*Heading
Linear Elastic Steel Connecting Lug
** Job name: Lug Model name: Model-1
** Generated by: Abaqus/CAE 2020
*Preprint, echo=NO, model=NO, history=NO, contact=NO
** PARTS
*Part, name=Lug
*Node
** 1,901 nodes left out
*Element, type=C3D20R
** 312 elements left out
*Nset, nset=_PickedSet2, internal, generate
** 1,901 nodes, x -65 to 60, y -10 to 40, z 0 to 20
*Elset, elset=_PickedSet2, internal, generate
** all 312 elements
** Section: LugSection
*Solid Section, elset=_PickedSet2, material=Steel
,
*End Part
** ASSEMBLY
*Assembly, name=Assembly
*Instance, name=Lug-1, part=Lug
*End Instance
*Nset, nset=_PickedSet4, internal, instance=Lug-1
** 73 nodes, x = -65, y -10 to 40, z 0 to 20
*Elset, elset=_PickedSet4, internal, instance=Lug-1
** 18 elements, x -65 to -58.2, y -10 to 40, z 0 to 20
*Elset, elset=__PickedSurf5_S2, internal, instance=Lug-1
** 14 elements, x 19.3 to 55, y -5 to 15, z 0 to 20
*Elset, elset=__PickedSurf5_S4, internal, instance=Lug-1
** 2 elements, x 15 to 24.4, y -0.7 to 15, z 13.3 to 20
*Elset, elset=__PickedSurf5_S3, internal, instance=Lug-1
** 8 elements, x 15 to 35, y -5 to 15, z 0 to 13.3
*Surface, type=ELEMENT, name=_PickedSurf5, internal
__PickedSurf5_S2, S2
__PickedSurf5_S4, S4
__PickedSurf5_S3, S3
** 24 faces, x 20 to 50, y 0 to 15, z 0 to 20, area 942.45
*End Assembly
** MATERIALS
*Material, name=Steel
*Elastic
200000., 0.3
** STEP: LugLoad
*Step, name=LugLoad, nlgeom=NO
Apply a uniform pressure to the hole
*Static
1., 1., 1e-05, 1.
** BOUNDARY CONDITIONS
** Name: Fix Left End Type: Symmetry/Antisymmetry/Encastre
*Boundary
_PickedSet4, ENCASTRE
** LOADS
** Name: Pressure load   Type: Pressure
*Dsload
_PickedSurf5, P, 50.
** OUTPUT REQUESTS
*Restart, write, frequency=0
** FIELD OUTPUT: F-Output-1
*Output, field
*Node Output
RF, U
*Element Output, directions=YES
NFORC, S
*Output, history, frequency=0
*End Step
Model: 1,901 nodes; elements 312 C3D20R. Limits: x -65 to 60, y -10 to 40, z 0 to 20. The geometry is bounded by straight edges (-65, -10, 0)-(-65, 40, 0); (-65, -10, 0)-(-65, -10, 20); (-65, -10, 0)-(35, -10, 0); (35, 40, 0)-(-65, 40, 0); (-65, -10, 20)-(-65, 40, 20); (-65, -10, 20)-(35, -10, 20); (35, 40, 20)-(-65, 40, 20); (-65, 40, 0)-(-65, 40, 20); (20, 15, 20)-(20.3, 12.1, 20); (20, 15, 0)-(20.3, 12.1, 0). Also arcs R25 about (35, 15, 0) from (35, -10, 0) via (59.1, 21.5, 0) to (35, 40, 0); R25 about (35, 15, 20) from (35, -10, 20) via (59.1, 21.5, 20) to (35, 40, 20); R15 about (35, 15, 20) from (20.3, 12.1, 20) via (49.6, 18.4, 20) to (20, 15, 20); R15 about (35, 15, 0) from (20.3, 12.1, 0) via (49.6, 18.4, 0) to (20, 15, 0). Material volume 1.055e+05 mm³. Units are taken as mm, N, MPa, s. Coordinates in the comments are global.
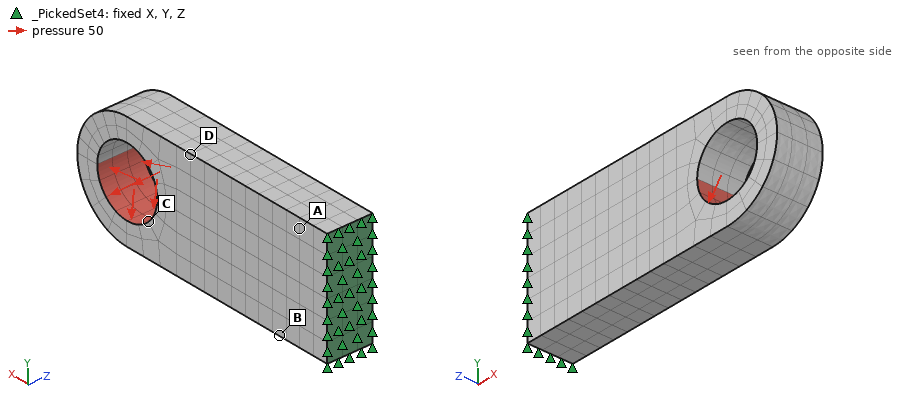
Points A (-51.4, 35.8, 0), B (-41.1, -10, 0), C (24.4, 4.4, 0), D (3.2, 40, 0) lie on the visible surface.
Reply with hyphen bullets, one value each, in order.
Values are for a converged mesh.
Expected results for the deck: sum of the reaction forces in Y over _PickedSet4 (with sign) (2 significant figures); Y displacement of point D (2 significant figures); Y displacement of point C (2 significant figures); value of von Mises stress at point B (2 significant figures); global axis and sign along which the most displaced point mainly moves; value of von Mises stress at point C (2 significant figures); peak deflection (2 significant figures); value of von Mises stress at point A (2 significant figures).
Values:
- 30000 N
- -0.16 mm
- -0.25 mm
- 270 MPa
- -Y
- 310 MPa
- 0.42 mm
- 250 MPa
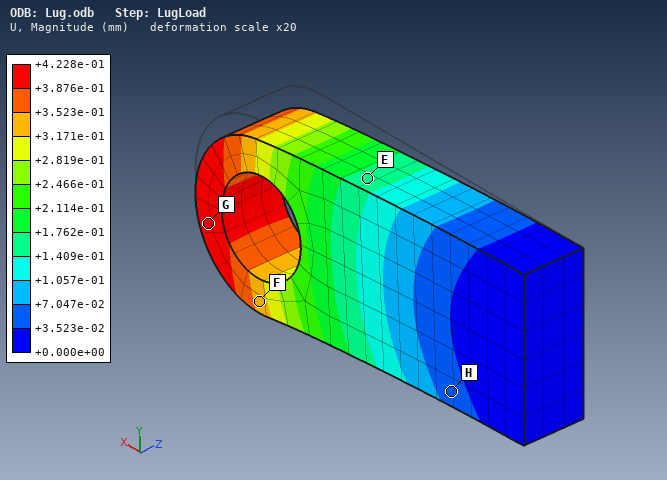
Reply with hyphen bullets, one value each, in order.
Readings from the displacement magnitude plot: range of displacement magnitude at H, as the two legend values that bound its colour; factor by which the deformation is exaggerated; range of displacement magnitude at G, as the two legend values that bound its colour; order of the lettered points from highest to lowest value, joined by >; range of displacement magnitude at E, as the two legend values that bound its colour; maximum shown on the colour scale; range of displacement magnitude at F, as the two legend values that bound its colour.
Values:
- +3.523e-02 to +7.047e-02 mm
- 20
- +3.876e-01 to +4.228e-01 mm
- G > F > E > H
- +1.409e-01 to +1.762e-01 mm
- +4.228e-01 mm
- +3.171e-01 to +3.523e-01 mm
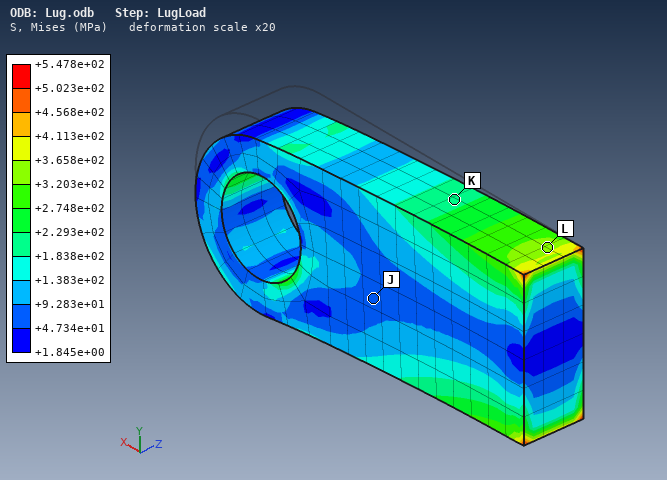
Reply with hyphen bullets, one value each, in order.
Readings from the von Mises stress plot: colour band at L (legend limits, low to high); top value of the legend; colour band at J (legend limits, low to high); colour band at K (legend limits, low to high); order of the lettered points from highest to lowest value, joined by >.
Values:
- +3.203e+02 to +3.658e+02 MPa
- +5.478e+02 MPa
- +4.734e+01 to +9.283e+01 MPa
- +1.838e+02 to +2.293e+02 MPa
- L > K > J
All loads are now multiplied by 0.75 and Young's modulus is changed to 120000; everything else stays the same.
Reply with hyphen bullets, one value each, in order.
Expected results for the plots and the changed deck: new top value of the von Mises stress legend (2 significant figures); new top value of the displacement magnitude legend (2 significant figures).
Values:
- 410 MPa
- 0.53 mm
